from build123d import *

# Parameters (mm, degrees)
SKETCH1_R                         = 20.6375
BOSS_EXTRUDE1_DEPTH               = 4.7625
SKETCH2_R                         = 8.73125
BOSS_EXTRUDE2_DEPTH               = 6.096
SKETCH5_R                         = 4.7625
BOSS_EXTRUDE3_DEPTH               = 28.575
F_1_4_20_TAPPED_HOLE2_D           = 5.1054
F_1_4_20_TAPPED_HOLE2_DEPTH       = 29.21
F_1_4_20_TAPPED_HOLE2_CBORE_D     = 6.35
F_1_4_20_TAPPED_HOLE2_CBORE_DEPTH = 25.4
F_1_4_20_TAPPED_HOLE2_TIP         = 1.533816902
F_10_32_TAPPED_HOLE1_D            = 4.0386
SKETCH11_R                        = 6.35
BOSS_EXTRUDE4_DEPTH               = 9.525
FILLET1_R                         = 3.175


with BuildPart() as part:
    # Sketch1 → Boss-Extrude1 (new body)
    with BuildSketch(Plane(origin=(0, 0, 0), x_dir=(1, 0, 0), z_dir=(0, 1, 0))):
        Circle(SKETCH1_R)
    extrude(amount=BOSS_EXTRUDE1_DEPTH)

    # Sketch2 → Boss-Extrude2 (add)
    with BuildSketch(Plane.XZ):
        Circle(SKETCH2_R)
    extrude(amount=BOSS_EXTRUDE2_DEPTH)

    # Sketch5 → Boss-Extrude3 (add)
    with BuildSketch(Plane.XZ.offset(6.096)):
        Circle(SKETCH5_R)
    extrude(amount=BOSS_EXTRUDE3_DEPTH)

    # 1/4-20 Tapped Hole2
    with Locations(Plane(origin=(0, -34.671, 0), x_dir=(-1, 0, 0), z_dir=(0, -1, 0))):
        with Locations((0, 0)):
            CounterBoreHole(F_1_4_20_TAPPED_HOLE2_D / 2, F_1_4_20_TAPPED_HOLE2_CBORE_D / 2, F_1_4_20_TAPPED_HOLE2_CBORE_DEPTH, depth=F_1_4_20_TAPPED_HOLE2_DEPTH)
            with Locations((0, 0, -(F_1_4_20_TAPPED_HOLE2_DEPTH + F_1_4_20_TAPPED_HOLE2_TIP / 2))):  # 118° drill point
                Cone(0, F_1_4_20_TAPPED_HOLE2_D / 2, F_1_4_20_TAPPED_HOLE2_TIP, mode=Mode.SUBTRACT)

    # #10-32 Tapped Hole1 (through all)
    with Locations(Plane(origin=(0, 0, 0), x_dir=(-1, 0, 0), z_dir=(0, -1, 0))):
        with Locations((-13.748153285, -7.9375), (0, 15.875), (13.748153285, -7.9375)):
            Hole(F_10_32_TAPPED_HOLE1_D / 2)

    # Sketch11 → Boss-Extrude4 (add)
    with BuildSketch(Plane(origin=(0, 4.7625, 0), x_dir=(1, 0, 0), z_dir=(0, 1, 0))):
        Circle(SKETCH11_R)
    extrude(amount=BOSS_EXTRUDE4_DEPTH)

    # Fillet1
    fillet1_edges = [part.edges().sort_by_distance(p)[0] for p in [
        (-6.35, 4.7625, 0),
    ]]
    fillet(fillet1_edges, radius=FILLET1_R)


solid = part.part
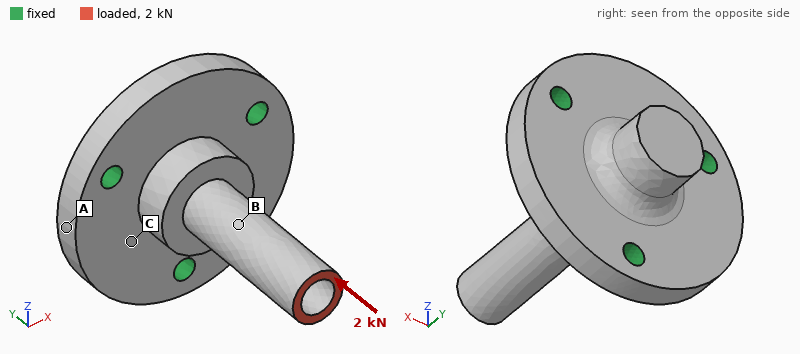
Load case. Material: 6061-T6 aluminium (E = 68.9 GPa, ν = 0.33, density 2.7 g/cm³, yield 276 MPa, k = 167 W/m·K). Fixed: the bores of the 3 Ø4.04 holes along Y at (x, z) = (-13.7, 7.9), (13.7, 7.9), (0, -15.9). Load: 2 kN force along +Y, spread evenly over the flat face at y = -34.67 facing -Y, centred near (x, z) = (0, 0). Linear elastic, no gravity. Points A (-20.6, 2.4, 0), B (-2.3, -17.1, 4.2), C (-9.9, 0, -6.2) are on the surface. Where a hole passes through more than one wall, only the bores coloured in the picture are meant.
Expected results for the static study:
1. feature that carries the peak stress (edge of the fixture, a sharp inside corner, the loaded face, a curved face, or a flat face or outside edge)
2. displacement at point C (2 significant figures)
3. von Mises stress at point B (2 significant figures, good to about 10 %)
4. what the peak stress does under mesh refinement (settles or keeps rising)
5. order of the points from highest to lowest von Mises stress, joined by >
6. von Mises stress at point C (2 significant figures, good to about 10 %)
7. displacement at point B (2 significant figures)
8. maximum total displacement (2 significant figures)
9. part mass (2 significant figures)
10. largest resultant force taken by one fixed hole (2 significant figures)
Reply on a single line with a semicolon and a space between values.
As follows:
edge of the fixture; 5.8 µm; 51 MPa; keeps rising; B > C > A; 13 MPa; 16 µm; 29 µm; 27 g; 670 N
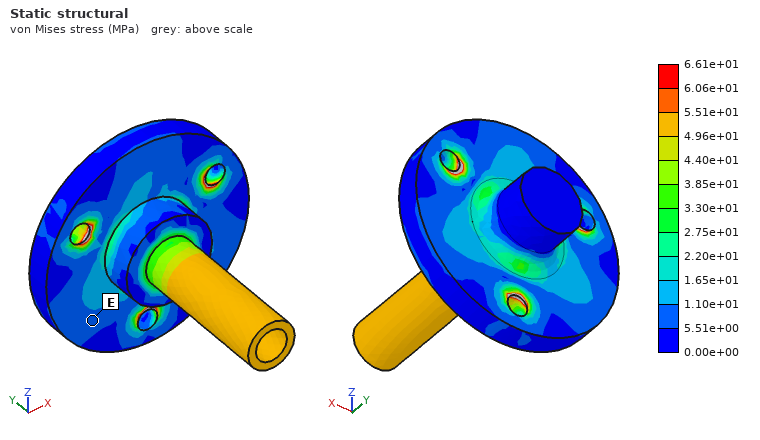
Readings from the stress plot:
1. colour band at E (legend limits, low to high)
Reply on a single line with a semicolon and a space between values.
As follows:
5.51e+00 to 1.10e+01 MPa
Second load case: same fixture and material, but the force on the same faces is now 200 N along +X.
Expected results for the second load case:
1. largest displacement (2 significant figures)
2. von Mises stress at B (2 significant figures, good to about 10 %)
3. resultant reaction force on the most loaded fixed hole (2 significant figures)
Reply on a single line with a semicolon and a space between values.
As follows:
0.11 mm; 28 MPa; 290 N
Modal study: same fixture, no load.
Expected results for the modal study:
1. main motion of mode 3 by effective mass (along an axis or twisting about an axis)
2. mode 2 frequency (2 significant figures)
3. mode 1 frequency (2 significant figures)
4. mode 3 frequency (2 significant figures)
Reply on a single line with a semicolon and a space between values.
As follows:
along Y; 7400 Hz; 7400 Hz; 19 kHz
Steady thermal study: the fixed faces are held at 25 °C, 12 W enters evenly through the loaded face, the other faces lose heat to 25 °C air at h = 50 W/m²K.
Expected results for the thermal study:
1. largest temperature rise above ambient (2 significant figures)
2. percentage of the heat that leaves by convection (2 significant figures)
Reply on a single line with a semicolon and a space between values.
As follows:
51 K; 18 %
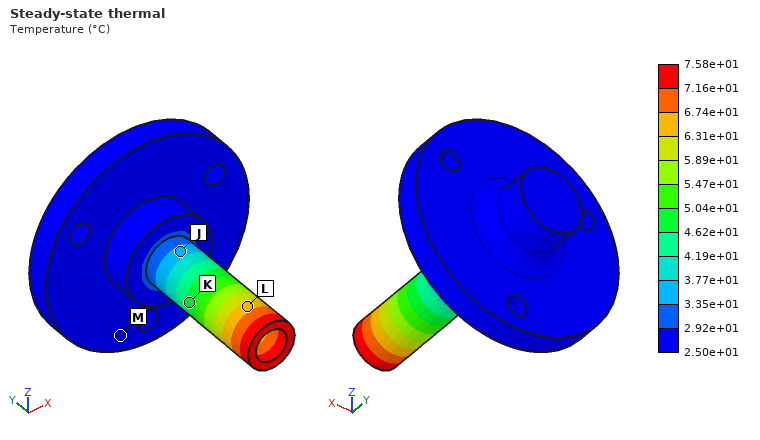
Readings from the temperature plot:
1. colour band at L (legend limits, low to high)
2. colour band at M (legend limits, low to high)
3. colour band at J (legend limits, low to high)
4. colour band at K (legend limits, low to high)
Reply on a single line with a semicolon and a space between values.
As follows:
6.31e+01 to 6.74e+01 °C; 2.50e+01 to 2.92e+01 °C; 3.35e+01 to 3.77e+01 °C; 4.62e+01 to 5.04e+01 °C
